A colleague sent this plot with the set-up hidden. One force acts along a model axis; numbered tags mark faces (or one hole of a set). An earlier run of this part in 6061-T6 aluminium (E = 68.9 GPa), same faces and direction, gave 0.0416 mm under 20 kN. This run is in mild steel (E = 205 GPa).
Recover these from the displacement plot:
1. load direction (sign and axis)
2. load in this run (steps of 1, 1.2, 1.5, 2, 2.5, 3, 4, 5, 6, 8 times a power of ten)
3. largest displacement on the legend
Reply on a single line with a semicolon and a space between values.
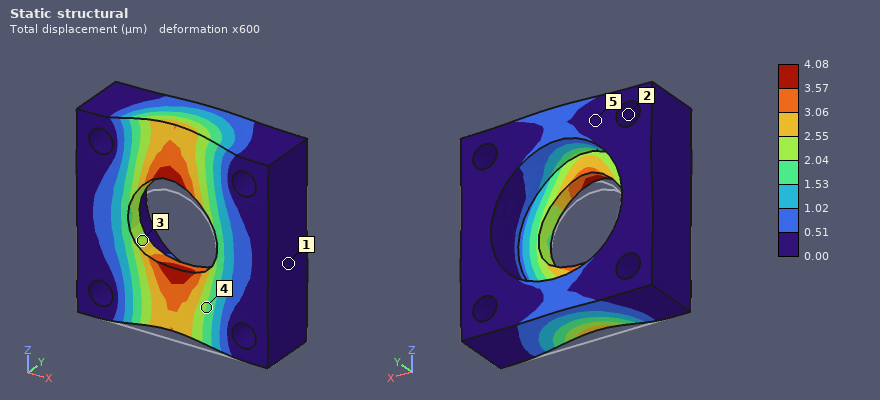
+Z; 6 kN; 4.08 µm
